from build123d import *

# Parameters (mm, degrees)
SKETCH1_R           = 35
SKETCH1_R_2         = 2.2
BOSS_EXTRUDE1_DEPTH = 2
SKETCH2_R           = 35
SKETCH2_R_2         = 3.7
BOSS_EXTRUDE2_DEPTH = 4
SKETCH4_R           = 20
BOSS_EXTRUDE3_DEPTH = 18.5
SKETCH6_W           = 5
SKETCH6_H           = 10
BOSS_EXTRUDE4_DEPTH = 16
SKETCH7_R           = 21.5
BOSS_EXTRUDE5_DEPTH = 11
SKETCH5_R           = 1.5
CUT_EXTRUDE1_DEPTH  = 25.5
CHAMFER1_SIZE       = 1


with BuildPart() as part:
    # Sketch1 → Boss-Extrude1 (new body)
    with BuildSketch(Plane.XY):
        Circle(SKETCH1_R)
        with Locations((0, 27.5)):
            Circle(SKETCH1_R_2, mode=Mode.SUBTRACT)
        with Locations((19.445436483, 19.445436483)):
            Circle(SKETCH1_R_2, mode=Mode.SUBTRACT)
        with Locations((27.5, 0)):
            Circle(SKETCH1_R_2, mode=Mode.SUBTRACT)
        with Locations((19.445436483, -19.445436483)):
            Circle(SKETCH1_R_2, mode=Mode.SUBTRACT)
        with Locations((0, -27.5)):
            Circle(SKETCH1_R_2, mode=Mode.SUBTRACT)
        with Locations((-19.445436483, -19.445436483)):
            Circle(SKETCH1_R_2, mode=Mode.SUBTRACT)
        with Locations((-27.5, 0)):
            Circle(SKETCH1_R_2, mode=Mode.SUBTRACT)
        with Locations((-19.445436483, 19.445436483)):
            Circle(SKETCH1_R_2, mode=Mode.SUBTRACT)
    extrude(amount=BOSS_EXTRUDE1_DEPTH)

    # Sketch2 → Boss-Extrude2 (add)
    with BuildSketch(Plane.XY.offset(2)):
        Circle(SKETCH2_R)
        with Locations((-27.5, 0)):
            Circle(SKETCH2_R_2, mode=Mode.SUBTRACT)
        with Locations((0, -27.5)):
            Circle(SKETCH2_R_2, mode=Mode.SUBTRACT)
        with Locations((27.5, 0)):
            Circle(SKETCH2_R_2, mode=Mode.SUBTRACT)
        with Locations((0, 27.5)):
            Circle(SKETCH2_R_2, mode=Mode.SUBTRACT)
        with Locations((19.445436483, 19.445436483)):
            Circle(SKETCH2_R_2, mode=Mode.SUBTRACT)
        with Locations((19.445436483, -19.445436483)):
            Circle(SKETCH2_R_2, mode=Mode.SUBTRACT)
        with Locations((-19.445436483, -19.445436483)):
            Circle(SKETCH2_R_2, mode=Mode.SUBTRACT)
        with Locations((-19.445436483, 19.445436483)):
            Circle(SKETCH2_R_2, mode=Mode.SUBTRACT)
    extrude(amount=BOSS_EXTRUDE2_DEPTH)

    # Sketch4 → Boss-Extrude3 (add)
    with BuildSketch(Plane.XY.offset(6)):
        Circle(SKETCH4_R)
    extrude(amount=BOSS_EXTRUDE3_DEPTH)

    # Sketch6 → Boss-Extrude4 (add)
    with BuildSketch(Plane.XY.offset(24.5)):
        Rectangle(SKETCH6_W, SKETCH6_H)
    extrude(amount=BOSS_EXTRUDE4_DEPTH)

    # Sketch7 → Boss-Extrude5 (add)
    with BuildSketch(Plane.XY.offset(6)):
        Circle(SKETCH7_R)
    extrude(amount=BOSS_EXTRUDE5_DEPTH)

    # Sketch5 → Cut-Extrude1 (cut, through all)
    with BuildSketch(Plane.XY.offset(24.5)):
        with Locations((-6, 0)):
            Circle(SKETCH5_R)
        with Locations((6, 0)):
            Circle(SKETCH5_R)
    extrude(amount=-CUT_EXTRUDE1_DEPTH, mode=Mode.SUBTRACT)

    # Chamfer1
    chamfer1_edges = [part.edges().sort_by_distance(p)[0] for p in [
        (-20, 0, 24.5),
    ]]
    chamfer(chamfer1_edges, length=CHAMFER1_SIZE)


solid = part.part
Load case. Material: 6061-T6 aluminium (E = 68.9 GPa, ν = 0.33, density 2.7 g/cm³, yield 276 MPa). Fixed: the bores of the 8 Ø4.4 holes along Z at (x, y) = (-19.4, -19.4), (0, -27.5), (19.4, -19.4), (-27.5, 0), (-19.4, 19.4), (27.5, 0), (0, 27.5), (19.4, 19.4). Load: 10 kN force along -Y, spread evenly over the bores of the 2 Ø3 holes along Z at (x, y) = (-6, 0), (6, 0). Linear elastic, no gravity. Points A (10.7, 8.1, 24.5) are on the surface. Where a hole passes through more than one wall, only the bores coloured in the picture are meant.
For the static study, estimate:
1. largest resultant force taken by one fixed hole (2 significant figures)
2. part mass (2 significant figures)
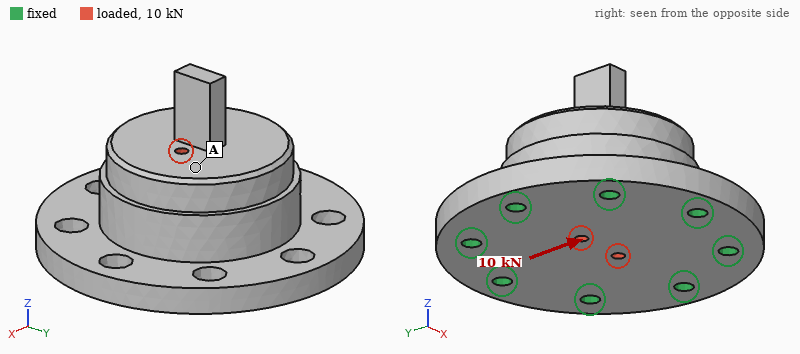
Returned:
2.1 kN
130 g
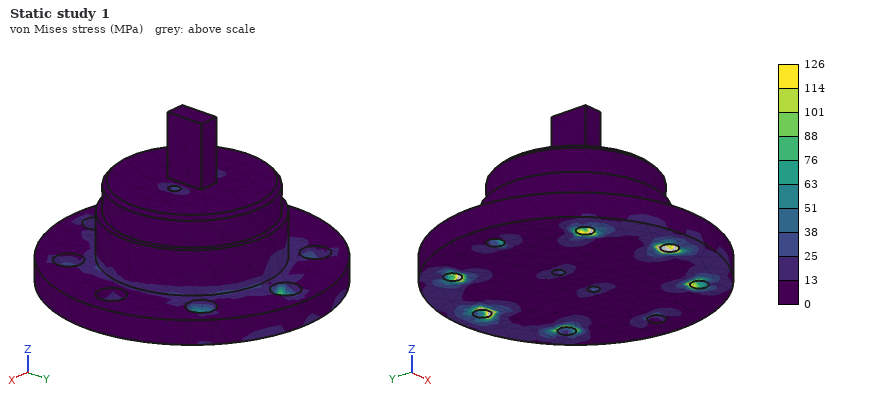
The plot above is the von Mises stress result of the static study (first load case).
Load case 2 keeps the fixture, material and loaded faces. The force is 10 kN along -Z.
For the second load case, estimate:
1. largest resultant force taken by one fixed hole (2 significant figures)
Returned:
1.7 kN
